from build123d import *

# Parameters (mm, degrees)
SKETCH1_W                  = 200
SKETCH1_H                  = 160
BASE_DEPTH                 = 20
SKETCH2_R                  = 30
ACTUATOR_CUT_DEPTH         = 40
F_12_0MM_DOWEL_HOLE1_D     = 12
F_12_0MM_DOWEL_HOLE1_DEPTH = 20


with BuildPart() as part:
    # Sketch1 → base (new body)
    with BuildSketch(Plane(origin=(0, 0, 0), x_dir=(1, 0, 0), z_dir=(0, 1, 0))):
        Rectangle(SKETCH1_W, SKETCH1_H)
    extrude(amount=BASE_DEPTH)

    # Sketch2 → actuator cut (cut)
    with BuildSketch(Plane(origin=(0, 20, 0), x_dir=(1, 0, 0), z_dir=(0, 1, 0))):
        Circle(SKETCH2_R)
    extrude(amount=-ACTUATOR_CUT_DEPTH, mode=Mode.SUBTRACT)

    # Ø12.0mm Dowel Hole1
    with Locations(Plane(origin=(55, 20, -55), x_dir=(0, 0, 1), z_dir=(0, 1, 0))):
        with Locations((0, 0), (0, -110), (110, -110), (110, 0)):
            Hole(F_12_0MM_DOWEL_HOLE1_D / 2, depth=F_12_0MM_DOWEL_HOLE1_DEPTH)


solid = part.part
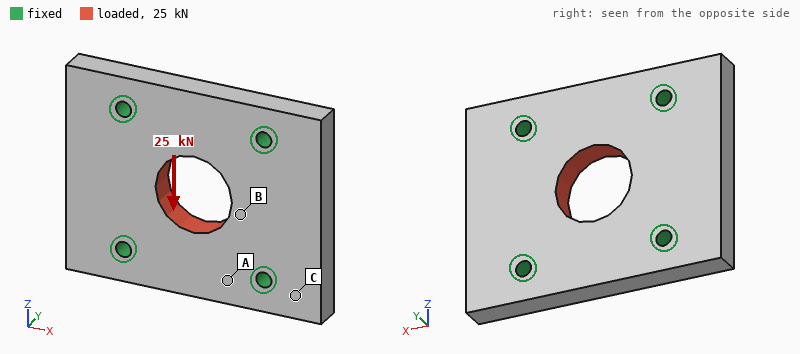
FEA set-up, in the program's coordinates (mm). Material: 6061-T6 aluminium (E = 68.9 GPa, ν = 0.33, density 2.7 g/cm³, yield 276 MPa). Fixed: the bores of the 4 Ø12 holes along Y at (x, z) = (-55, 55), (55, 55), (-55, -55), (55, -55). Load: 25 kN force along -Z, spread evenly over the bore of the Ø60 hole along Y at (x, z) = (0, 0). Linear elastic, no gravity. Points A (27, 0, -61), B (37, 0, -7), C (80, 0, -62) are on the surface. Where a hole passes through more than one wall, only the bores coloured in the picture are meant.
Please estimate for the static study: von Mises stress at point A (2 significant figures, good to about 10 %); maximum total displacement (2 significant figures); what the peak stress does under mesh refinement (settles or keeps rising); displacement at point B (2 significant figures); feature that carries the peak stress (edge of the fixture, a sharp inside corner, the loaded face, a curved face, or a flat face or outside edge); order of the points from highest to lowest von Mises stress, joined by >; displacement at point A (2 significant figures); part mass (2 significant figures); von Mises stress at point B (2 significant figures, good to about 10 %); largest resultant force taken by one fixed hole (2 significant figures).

5.1 MPa
9.7 µm
keeps rising
5.2 µm
edge of the fixture
B > A > C
5.4 µm
1.6 kg
9.3 MPa
6.6 kN
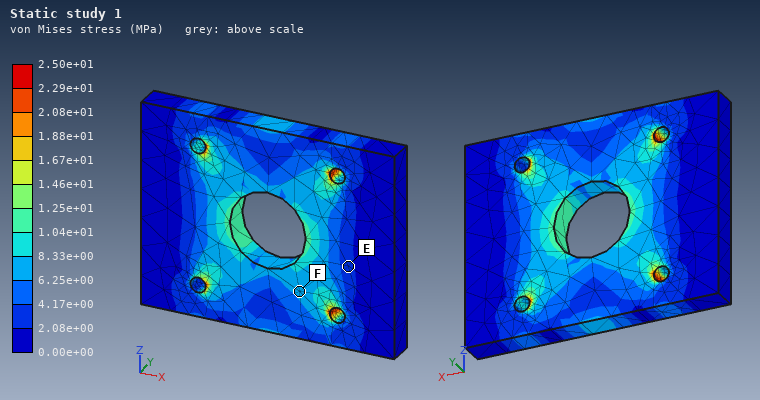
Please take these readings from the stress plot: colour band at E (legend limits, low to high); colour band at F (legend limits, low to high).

2.08e+00 to 4.17e+00 MPa
6.25e+00 to 8.33e+00 MPa
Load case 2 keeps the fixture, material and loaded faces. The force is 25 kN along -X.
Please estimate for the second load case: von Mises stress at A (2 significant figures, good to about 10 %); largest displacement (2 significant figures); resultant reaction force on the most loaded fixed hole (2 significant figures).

3.3 MPa
8.2 µm
6.4 kN
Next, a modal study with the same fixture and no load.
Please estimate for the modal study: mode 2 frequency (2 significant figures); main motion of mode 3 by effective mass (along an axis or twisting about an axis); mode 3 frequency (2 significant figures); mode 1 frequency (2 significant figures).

5100 Hz
along Y
6100 Hz
5000 Hz
